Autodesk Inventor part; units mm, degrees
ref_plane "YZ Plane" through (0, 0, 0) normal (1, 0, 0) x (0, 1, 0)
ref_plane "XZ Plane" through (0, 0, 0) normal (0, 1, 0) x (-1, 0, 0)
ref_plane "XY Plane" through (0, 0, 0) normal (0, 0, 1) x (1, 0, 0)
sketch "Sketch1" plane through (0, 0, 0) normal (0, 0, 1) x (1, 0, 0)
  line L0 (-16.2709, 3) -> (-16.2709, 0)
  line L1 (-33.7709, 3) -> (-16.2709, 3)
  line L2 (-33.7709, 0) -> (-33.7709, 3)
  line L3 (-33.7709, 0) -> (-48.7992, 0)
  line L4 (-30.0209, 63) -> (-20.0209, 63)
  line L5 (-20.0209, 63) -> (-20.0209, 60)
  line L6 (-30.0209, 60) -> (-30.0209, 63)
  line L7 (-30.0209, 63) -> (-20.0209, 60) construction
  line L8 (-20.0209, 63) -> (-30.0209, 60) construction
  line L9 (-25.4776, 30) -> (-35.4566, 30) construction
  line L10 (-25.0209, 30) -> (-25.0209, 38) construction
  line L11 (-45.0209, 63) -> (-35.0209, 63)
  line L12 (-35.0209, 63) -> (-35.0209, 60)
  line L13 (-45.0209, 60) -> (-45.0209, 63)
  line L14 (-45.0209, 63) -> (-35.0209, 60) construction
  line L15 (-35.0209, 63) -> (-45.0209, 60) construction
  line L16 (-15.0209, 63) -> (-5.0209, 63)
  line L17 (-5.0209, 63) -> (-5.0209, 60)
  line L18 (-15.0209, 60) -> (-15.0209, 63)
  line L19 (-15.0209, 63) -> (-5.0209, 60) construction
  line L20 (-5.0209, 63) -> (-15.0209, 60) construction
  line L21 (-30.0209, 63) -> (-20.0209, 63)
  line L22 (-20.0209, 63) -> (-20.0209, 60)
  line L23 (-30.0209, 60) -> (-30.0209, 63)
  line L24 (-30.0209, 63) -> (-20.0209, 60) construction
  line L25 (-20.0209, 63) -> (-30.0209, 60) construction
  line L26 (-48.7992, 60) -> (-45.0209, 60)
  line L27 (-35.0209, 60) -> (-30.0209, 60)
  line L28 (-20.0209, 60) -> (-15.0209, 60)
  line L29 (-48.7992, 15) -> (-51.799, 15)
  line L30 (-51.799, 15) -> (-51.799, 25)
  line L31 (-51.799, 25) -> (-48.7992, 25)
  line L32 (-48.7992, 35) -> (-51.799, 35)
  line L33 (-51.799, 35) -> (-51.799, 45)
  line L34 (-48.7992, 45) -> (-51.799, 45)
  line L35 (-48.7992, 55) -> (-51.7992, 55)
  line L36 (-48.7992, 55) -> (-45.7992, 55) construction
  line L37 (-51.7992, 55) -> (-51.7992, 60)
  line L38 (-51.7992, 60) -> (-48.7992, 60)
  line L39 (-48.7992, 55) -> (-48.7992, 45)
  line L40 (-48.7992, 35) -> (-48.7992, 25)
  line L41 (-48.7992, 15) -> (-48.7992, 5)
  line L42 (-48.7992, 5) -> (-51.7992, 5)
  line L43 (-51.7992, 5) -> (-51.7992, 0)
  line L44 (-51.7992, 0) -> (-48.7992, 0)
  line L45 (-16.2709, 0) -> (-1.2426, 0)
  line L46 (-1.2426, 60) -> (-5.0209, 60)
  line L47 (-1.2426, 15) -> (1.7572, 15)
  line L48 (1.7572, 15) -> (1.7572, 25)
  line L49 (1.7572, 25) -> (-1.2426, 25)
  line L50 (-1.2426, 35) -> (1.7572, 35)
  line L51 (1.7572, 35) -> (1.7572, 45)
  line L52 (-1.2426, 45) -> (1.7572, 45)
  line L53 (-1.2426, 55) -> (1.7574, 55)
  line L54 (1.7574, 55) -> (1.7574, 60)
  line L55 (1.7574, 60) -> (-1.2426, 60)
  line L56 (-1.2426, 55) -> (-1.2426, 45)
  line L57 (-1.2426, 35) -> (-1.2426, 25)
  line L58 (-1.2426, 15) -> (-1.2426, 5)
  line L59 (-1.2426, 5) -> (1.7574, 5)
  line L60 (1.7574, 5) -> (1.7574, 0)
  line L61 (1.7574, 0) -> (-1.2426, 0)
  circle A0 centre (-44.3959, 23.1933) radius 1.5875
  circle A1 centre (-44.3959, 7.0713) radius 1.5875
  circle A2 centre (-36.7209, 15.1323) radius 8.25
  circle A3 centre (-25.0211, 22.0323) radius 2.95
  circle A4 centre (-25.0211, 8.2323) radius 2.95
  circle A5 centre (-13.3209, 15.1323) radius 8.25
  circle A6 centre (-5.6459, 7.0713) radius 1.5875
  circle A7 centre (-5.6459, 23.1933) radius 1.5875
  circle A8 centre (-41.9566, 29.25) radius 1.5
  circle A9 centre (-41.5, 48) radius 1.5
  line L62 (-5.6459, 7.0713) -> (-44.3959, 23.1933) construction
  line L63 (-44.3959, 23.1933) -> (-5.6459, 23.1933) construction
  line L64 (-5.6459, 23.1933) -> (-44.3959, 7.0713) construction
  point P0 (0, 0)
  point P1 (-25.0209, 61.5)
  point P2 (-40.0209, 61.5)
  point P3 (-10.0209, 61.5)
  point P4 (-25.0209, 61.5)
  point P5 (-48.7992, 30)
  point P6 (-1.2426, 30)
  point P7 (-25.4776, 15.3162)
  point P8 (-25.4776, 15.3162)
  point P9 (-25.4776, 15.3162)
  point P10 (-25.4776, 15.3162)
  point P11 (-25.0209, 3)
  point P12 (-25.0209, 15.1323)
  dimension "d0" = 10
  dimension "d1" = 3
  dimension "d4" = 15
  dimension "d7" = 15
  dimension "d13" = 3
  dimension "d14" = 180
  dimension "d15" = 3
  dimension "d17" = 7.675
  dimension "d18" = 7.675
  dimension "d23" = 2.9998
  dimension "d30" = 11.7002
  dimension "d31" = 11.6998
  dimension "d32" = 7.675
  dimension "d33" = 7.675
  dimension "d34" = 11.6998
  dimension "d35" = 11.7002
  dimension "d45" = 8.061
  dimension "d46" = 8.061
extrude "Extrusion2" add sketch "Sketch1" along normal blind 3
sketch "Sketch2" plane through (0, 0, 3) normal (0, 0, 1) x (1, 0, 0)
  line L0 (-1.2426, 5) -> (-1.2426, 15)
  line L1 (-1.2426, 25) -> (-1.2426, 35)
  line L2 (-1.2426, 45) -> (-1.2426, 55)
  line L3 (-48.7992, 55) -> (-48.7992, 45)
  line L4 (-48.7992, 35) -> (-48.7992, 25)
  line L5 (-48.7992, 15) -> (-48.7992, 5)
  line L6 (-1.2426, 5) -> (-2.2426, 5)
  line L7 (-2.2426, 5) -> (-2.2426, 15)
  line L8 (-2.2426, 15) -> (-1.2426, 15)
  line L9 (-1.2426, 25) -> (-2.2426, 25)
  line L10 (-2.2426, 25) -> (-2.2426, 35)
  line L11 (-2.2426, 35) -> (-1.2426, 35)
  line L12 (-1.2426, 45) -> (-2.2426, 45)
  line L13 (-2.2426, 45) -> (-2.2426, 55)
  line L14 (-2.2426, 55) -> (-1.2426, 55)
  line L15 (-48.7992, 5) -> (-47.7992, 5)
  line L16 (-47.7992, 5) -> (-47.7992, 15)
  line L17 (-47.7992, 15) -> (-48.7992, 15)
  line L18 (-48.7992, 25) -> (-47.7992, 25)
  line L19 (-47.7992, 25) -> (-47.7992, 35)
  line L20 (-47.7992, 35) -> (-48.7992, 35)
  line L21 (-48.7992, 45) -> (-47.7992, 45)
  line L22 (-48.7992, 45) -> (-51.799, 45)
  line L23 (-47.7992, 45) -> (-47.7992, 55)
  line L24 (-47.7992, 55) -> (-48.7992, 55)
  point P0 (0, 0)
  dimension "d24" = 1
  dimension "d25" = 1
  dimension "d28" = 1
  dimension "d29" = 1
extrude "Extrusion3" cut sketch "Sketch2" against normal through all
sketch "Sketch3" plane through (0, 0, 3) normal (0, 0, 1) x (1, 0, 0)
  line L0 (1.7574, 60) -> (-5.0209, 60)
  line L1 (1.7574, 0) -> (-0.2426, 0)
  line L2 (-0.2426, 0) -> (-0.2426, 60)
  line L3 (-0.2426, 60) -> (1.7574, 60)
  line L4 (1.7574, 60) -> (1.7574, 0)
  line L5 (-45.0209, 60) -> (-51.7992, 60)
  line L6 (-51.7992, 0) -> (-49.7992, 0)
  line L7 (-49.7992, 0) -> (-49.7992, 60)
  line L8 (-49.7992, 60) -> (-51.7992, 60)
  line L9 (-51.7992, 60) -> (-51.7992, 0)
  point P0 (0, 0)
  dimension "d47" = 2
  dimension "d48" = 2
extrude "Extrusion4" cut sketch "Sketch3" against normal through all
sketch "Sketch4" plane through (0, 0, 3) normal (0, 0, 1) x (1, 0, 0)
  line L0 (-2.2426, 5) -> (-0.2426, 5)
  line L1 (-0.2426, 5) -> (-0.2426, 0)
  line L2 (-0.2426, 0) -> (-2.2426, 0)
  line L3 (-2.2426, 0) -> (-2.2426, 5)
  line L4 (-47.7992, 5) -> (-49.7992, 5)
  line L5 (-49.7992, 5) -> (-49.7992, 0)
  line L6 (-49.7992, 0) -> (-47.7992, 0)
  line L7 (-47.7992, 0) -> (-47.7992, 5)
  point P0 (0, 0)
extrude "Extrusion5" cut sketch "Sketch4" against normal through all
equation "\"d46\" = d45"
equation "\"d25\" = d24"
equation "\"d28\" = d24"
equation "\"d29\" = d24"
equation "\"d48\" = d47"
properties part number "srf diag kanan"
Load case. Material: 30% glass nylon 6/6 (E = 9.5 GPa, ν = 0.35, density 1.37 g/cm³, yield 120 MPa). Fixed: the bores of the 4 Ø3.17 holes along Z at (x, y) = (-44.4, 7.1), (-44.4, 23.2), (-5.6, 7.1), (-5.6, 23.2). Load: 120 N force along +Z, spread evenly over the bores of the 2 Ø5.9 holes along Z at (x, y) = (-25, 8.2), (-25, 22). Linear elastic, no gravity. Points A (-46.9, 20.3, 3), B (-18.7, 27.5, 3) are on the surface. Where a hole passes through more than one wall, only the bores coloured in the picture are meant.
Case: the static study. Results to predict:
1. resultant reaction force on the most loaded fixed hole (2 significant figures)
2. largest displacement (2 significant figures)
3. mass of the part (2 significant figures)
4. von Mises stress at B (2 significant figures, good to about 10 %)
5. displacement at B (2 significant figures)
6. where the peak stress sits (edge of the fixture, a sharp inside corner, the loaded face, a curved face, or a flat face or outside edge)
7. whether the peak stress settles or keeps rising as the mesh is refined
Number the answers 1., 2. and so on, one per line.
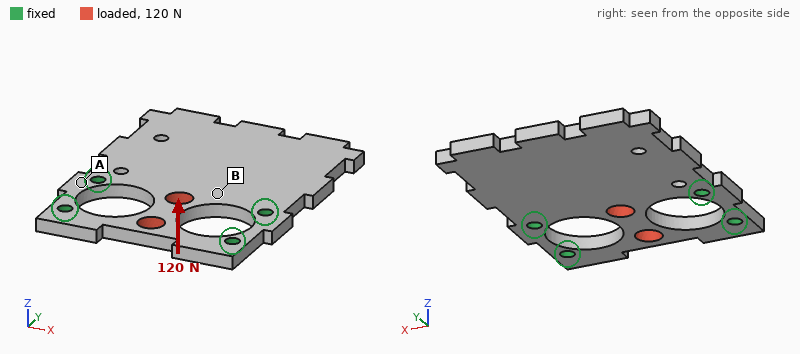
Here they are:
1. 31 N
2. 0.14 mm
3. 9.6 g
4. 10 MPa
5. 0.054 mm
6. edge of the fixture
7. keeps rising
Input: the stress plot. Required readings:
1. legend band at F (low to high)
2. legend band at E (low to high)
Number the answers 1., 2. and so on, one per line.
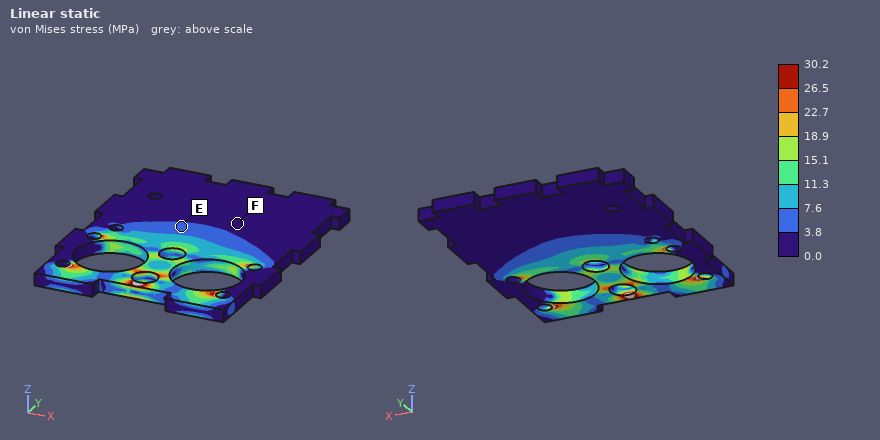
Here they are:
1. 0.0 to 3.8 MPa
2. 3.8 to 7.6 MPa
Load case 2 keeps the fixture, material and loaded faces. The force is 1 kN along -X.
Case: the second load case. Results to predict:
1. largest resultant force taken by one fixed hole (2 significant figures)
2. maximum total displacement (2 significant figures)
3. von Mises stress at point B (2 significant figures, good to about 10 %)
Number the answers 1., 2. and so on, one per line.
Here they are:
1. 280 N
2. 65 µm
3. 5.8 MPa
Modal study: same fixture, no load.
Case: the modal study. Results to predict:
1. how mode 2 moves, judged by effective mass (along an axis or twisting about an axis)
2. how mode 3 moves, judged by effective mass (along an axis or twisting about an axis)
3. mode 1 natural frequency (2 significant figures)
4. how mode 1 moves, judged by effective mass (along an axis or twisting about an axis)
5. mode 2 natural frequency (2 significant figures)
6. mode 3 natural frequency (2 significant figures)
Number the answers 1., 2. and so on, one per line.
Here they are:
1. twisting about Y
2. along Z
3. 670 Hz
4. along Z
5. 1700 Hz
6. 4000 Hz
